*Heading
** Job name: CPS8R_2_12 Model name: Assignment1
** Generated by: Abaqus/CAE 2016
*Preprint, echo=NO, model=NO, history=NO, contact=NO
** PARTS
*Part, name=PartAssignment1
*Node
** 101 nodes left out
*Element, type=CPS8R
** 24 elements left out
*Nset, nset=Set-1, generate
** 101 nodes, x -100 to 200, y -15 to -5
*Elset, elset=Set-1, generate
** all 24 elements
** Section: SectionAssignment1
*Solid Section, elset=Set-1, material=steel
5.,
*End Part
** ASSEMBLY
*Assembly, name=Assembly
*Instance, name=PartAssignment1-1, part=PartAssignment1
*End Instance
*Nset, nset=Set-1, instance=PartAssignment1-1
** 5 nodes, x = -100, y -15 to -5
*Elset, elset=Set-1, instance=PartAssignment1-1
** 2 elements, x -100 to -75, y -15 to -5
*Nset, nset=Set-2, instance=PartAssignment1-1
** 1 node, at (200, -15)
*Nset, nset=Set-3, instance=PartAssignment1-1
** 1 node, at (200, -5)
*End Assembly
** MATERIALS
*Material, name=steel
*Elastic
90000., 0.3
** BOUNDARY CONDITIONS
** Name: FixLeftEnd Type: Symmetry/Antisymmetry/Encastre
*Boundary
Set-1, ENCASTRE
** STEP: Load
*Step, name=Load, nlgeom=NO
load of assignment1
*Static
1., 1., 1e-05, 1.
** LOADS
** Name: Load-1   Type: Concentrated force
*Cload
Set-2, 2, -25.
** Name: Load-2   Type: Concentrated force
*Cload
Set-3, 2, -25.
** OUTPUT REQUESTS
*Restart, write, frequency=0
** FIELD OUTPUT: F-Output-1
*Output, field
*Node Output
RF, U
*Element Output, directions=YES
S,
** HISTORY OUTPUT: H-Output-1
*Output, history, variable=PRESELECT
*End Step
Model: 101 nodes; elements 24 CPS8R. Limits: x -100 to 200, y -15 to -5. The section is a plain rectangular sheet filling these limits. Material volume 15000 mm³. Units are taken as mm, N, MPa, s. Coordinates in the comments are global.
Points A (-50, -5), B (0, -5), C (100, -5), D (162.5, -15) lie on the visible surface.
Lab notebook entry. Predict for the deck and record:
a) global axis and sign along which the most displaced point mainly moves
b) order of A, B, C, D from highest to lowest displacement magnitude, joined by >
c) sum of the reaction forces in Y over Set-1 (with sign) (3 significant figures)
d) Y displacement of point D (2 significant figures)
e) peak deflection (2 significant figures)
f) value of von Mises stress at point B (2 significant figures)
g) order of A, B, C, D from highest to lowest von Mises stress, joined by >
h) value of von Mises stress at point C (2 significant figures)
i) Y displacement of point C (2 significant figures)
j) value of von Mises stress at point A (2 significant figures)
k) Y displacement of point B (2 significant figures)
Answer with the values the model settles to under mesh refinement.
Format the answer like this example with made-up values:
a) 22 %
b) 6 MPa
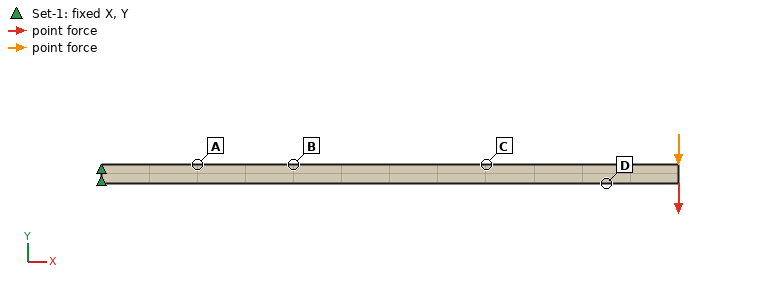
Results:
a) -Y
b) D > C > B > A
c) 50.0 N
d) -9.7 mm
e) 12 mm
f) 120 MPa
g) A > B > C > D
h) 59 MPa
i) -6.2 mm
j) 150 MPa
k) -1.8 mm
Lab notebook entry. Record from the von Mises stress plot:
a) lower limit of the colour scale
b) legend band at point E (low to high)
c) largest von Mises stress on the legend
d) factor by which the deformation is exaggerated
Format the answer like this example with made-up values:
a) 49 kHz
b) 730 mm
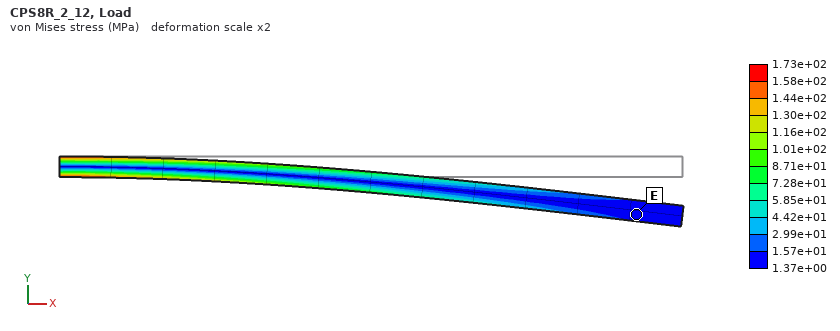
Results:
a) 1.37e+00 MPa
b) 1.37e+00 to 1.57e+01 MPa
c) 1.73e+02 MPa
d) 2
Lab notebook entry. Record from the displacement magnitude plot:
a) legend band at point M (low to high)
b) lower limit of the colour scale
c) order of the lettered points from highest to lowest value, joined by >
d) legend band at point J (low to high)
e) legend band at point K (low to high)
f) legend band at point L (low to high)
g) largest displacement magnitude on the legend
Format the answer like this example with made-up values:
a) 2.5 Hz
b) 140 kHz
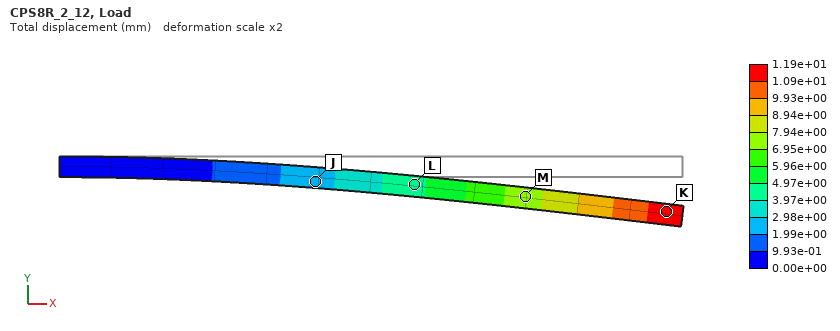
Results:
a) 6.95e+00 to 7.94e+00 mm
b) 0.00e+00 mm
c) K > M > L > J
d) 1.99e+00 to 2.98e+00 mm
e) 1.09e+01 to 1.19e+01 mm
f) 3.97e+00 to 4.97e+00 mm
g) 1.19e+01 mm
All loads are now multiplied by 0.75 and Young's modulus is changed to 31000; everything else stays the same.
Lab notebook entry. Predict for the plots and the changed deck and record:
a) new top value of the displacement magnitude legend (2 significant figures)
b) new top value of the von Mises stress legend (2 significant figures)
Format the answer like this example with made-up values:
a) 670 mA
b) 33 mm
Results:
a) 26 mm
b) 130 MPa
